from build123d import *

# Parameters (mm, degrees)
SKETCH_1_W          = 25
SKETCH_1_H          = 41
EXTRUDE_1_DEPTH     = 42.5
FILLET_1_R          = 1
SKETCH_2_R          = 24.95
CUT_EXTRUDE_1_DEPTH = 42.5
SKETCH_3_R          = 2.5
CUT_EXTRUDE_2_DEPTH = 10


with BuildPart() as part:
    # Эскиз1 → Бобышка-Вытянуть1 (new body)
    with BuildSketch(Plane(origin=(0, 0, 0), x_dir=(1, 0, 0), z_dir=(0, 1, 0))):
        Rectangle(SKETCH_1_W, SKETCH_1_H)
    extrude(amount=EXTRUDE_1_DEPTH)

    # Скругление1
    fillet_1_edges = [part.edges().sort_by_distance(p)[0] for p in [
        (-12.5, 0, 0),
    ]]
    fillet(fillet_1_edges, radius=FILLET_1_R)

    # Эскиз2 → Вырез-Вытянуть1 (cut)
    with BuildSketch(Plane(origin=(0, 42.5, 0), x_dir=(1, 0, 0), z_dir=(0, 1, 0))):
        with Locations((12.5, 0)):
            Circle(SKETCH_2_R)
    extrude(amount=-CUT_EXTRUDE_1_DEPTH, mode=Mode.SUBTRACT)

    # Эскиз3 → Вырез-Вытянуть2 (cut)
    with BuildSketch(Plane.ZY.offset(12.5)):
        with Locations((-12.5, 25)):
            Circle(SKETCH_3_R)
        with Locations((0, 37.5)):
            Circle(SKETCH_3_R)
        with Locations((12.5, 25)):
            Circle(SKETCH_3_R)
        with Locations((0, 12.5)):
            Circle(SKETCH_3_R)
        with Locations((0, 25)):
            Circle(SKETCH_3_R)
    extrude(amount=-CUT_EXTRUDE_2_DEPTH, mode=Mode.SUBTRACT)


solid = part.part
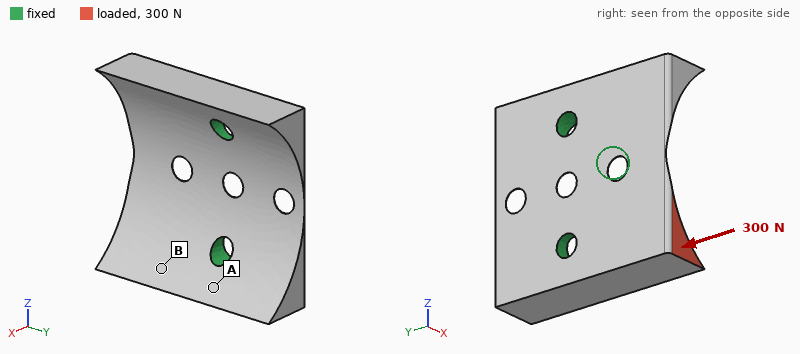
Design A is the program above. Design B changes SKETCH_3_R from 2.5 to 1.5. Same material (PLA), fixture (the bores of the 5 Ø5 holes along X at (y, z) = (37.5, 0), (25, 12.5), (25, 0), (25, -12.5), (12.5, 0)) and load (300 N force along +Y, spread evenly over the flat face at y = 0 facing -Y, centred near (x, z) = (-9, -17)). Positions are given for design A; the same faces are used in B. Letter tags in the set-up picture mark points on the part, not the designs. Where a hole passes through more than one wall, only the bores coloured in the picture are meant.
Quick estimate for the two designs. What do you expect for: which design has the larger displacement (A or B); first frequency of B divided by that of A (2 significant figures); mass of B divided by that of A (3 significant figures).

B
0.76
1.02
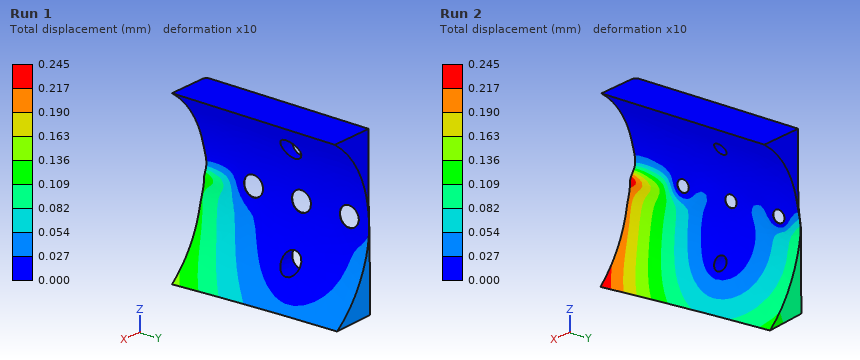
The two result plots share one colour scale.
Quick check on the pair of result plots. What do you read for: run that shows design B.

Run 2
